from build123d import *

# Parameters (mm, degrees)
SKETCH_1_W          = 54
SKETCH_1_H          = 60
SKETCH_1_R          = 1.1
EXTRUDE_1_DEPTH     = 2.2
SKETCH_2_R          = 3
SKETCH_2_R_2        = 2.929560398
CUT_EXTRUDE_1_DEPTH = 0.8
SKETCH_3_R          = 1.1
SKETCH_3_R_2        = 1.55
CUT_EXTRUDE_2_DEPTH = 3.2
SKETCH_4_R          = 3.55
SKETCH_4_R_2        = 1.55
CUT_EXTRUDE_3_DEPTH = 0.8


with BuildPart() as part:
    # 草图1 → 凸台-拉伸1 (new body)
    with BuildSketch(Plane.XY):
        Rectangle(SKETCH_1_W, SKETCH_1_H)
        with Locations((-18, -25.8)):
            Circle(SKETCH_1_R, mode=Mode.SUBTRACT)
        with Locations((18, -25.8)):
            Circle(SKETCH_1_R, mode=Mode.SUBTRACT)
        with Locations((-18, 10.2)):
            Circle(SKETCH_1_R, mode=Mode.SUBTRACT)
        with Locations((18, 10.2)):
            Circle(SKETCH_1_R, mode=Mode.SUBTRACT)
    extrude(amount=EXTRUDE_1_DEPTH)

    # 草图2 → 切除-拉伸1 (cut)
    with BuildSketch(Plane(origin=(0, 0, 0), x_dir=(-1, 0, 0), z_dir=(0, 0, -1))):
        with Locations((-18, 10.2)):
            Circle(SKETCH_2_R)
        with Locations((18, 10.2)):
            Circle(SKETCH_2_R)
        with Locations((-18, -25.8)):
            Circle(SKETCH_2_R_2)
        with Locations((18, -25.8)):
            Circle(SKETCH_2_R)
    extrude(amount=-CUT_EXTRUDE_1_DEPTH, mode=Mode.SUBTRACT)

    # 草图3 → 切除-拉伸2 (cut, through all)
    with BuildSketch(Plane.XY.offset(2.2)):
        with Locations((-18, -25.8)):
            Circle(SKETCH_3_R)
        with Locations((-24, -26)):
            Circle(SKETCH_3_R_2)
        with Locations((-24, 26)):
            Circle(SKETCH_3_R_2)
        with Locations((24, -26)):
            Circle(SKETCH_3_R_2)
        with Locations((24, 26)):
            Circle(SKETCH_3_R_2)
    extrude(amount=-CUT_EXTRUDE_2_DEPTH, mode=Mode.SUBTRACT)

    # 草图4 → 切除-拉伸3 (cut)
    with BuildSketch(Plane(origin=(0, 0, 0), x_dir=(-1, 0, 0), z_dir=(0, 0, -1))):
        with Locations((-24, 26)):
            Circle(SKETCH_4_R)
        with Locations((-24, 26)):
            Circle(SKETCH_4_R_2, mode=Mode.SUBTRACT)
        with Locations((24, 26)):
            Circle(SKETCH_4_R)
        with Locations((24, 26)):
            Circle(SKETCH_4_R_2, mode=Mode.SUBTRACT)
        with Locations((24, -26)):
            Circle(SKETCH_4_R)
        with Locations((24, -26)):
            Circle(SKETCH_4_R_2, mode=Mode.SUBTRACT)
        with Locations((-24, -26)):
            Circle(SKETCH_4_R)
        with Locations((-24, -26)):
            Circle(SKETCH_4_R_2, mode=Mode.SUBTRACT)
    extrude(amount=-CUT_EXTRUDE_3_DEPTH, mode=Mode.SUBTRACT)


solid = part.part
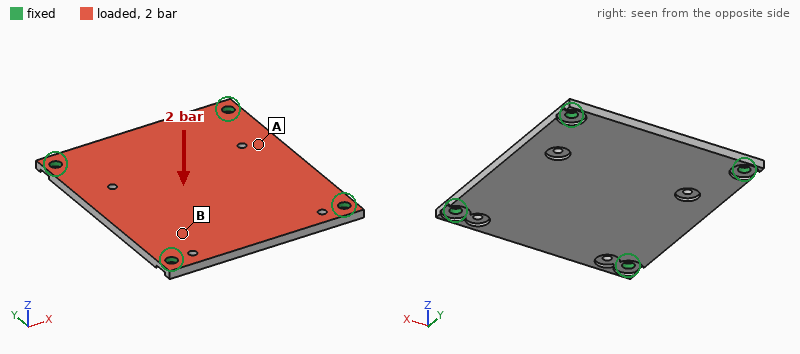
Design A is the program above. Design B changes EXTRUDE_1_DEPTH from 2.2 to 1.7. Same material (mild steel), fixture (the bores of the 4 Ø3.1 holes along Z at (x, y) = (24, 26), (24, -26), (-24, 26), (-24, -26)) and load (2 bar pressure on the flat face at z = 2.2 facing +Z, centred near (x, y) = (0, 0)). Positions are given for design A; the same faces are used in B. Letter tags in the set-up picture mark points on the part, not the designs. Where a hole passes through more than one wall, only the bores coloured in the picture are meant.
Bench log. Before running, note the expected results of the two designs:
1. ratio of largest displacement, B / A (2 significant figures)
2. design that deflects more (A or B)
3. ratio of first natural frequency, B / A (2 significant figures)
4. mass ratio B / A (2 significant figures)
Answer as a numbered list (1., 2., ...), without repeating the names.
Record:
1. 2.3
2. B
3. 0.75
4. 0.77
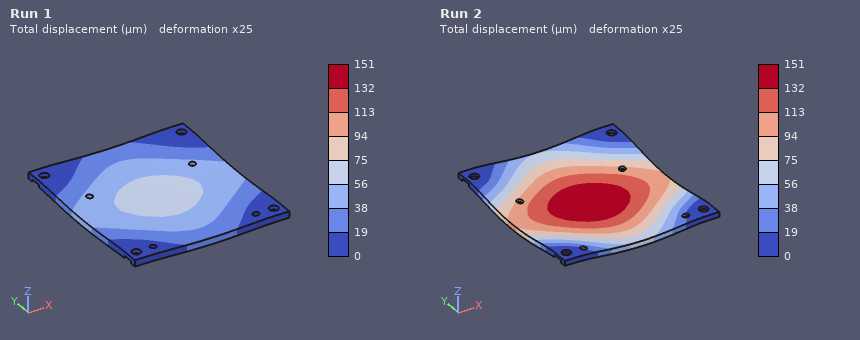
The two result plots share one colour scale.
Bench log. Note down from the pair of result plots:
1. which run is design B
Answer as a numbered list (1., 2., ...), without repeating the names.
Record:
1. Run 2
